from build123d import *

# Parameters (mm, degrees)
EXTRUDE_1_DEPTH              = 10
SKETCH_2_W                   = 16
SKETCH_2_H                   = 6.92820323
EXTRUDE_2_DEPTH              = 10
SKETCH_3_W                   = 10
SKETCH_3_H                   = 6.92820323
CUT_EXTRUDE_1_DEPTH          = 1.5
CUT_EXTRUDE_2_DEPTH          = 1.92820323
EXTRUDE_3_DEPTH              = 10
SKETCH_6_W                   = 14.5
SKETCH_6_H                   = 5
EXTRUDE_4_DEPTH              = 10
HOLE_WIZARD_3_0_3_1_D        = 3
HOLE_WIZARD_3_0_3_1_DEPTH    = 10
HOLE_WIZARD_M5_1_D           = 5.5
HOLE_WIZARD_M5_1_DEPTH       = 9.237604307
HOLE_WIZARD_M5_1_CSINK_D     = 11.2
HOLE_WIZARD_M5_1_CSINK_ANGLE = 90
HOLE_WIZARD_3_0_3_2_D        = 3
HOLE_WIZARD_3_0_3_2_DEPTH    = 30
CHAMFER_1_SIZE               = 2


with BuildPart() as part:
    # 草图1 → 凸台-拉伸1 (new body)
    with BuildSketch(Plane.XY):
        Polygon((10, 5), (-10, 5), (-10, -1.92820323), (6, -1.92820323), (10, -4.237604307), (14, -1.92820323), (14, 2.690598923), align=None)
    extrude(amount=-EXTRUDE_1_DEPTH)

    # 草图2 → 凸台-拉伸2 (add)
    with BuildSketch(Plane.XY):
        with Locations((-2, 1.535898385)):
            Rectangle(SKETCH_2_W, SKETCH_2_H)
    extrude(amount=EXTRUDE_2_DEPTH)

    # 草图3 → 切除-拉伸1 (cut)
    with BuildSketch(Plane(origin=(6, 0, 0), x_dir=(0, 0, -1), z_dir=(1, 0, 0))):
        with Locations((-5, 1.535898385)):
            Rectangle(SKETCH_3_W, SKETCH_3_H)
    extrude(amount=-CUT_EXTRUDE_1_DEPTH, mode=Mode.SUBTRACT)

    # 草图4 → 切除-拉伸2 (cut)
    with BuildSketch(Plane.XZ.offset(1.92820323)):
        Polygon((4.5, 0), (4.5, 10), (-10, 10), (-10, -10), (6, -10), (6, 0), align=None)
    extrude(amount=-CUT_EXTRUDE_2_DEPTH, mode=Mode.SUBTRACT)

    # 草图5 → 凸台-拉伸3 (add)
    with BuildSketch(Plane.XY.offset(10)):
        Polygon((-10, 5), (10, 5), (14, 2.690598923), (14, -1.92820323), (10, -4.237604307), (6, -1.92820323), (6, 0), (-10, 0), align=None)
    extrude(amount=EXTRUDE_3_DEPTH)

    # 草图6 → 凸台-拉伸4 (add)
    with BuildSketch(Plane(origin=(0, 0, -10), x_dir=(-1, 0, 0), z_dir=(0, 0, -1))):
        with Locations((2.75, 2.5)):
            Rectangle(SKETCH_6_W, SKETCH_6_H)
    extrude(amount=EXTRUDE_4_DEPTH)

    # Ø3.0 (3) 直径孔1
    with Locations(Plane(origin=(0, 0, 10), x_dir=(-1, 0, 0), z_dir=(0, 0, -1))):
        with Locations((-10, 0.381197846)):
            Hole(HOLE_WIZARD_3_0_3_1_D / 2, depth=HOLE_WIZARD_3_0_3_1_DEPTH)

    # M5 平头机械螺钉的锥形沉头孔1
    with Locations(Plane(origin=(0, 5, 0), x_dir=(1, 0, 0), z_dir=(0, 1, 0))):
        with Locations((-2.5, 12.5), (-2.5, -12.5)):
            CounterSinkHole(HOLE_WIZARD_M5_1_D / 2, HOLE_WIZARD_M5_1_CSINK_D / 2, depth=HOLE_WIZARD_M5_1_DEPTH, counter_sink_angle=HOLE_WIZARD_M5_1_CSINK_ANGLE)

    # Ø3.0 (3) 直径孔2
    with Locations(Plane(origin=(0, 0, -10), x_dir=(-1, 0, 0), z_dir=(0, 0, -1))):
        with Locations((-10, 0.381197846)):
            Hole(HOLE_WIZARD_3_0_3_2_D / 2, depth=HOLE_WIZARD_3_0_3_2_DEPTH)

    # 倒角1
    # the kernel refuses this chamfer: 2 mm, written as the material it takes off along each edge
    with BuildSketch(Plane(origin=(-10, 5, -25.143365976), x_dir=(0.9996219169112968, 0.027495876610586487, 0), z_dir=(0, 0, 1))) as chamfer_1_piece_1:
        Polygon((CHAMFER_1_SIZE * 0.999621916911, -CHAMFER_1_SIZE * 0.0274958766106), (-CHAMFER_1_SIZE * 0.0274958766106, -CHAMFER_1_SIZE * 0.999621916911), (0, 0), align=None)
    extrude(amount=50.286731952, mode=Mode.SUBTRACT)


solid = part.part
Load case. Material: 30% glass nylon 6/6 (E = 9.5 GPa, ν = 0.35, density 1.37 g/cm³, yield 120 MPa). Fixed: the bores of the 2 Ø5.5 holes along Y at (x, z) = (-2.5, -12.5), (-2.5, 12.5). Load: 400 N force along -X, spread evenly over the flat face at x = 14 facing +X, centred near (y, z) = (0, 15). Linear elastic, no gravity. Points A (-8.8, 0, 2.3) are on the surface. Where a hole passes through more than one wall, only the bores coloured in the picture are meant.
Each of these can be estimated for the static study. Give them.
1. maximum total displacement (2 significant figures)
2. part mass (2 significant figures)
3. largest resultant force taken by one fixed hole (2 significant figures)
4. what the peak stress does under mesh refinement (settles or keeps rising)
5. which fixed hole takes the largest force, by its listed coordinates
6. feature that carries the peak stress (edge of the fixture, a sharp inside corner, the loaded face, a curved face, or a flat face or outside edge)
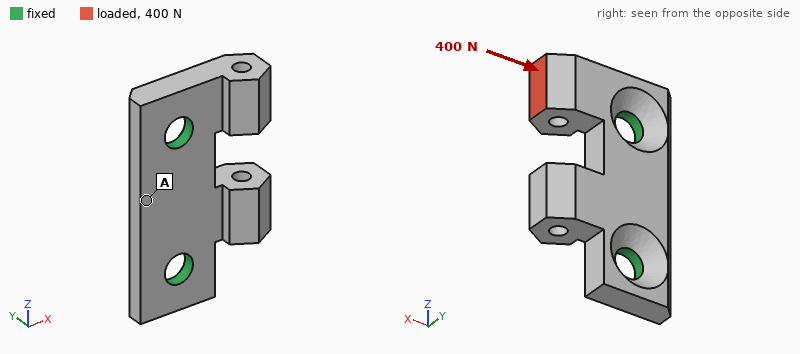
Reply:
0.11 mm
4.9 g
420 N
keeps rising
(-2.5, 12.5)
edge of the fixture
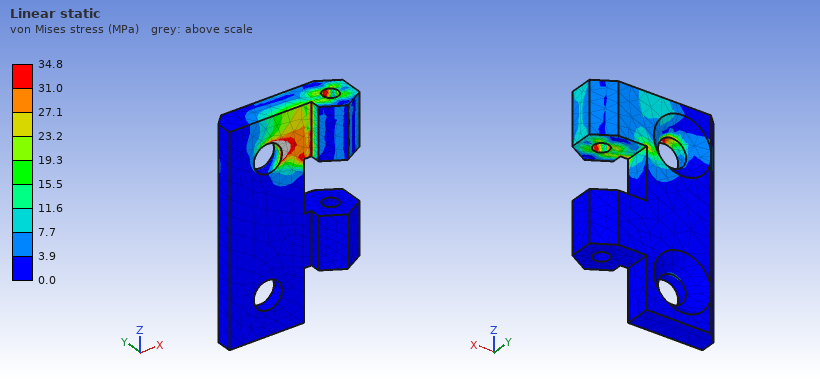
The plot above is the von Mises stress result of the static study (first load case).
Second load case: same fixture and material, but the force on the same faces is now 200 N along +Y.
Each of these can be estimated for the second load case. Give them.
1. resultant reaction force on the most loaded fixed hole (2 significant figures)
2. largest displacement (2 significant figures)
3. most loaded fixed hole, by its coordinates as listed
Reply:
220 N
0.44 mm
(-2.5, 12.5)
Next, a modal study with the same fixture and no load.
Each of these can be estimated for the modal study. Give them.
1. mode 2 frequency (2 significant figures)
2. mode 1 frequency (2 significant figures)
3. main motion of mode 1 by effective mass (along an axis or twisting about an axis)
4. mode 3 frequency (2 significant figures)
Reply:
5900 Hz
5300 Hz
along Y
11 kHz
